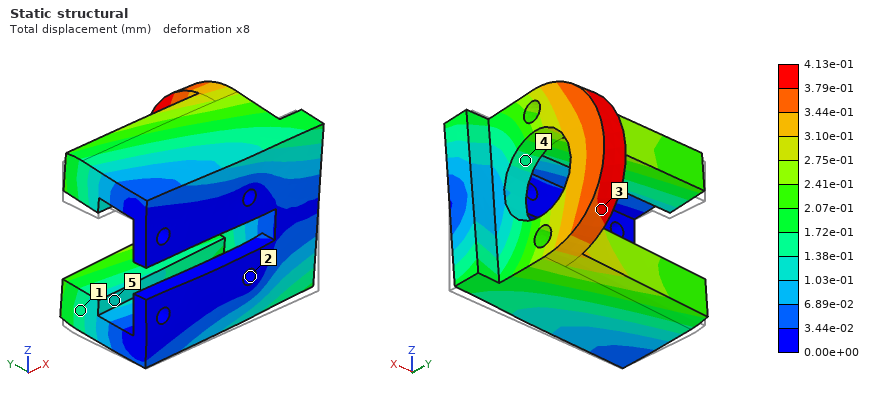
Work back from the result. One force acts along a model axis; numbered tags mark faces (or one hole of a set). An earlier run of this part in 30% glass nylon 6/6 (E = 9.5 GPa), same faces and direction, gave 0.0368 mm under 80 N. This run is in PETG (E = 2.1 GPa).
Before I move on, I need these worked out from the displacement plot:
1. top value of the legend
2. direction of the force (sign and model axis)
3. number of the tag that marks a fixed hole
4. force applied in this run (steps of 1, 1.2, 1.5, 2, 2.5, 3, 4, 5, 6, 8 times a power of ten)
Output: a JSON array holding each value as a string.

["4.13e-01 mm", "+Z", "2", "200 N"]
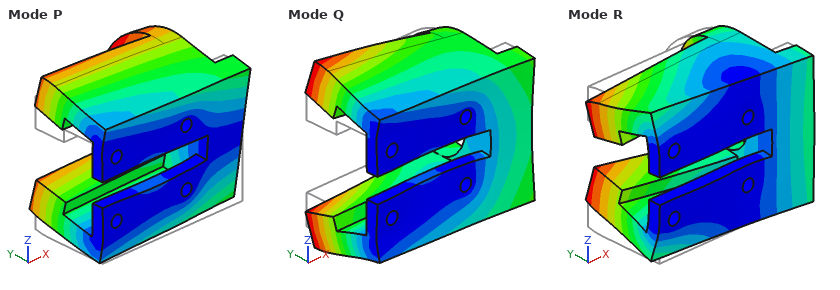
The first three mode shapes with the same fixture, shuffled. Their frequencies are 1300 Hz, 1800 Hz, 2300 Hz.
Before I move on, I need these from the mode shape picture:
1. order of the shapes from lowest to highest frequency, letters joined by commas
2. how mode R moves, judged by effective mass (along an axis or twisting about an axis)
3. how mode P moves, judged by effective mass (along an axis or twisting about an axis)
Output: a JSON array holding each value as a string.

["P, R, Q", "along X", "along Z"]
